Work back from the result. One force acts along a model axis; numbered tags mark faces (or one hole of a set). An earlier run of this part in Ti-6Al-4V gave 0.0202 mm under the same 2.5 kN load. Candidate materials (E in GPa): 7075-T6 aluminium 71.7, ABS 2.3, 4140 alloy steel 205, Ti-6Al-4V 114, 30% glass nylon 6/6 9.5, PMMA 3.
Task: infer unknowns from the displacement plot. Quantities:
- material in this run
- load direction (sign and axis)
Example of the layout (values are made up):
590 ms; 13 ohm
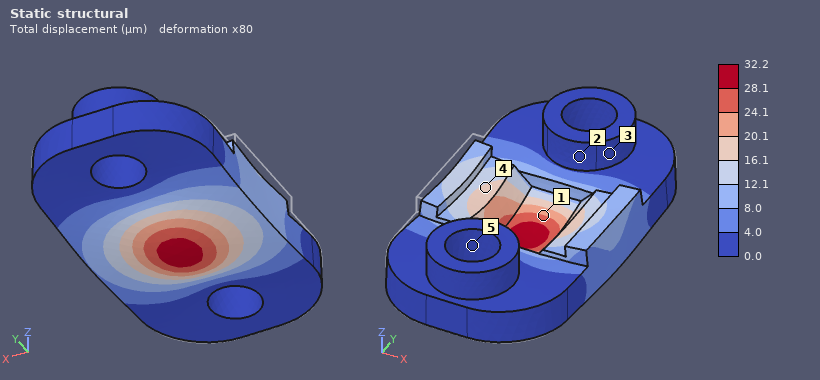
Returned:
7075-T6 aluminium; -Z
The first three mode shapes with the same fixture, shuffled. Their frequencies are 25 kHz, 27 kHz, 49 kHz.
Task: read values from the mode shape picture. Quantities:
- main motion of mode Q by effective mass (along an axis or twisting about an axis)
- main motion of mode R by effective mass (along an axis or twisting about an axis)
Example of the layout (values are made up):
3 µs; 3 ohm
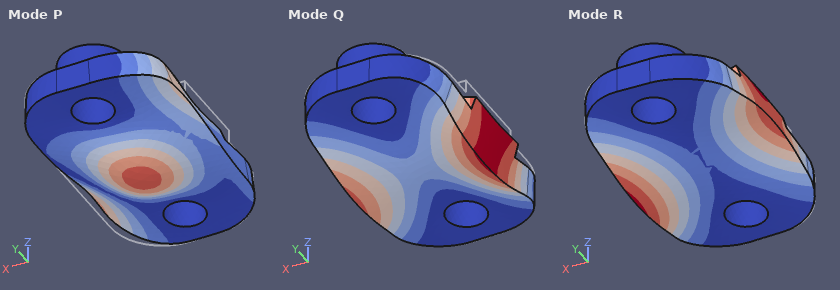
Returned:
along Z; twisting about Y
